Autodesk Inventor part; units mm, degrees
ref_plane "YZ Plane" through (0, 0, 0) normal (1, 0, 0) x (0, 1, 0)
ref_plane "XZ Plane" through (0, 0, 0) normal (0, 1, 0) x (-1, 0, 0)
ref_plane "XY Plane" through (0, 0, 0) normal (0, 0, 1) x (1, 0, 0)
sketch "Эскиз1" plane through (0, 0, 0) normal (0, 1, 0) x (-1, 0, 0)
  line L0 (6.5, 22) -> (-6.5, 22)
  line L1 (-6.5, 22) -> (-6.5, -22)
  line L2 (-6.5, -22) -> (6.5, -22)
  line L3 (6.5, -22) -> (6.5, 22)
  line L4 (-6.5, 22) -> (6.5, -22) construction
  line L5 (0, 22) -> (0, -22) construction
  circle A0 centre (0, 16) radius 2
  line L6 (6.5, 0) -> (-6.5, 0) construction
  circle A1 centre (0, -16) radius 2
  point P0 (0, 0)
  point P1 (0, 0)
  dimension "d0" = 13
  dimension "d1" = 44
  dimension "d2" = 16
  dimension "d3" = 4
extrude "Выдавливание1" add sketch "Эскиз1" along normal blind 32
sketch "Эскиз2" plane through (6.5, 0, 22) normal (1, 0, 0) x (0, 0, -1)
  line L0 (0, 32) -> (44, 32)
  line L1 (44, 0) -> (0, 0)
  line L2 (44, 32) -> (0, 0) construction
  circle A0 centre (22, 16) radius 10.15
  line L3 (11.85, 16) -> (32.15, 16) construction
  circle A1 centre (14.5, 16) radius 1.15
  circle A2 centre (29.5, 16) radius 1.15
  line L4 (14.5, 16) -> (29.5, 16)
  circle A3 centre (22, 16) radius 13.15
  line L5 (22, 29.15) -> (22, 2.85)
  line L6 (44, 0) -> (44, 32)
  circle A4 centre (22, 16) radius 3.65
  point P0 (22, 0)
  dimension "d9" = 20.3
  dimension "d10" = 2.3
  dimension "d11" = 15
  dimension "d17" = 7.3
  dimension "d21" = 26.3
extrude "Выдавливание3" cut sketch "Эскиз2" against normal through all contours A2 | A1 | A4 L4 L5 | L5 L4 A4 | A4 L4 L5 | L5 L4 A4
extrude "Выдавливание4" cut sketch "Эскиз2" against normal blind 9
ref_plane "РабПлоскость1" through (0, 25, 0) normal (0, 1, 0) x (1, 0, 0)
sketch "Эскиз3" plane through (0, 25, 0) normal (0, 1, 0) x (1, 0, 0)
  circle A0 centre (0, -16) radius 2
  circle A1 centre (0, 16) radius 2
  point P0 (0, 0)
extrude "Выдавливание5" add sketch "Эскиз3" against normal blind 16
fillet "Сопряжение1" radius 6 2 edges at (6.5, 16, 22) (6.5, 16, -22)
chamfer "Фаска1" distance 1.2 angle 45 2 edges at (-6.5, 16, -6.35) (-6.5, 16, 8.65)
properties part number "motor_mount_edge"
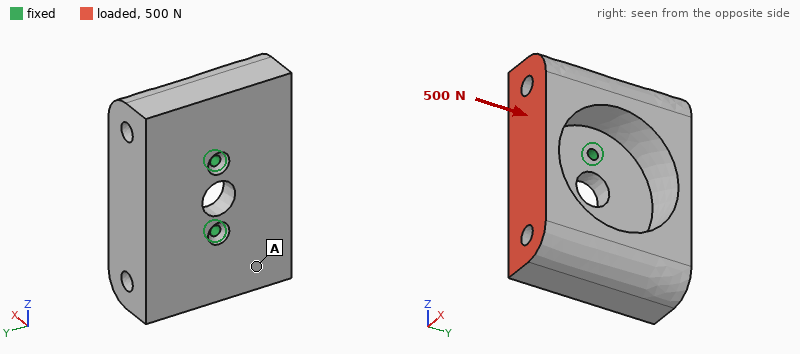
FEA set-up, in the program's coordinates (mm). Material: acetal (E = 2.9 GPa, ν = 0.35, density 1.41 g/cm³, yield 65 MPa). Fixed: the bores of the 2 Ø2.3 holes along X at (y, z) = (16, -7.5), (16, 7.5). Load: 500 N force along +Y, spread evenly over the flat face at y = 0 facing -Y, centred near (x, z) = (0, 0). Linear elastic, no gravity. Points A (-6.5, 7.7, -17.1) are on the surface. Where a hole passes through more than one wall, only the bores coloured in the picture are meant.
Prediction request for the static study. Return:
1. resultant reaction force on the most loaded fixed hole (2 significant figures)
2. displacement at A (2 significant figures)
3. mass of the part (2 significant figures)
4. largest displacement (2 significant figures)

250 N
0.19 mm
17 g
0.50 mm
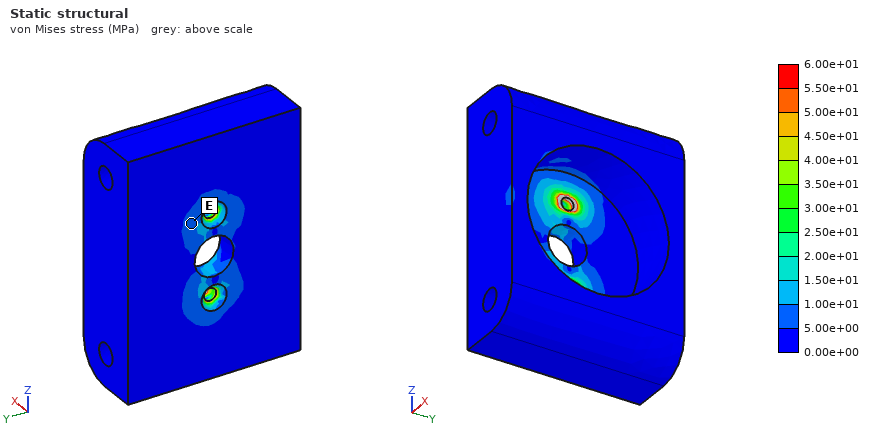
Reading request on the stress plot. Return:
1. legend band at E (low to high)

5.00e+00 to 1.00e+01 MPa
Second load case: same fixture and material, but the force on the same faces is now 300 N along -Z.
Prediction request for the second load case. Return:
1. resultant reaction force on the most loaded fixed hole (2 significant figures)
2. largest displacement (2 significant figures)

330 N
0.16 mm
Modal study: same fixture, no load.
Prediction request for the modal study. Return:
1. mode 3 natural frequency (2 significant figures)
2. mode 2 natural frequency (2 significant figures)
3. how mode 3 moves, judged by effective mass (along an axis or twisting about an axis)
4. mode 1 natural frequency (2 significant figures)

2800 Hz
1800 Hz
twisting about X
1000 Hz
